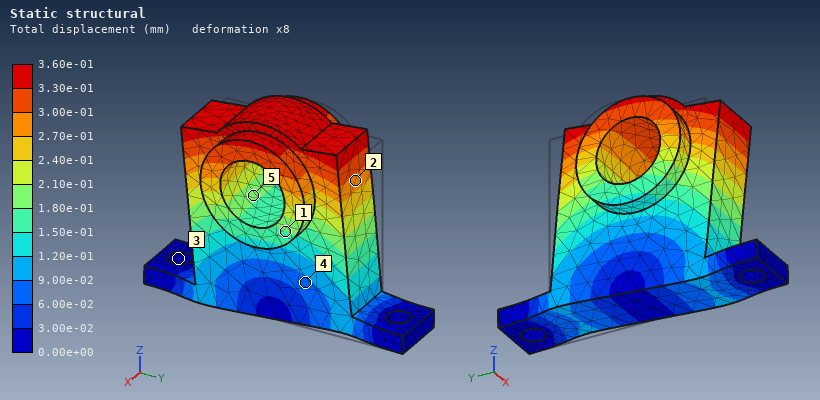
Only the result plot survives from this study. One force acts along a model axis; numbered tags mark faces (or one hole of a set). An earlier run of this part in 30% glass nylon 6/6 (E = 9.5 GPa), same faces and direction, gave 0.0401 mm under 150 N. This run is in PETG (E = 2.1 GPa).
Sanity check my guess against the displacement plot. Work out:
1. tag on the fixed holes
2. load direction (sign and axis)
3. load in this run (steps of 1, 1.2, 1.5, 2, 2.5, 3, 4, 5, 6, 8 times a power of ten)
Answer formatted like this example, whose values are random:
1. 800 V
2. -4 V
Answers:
1. 3
2. -Y
3. 300 N
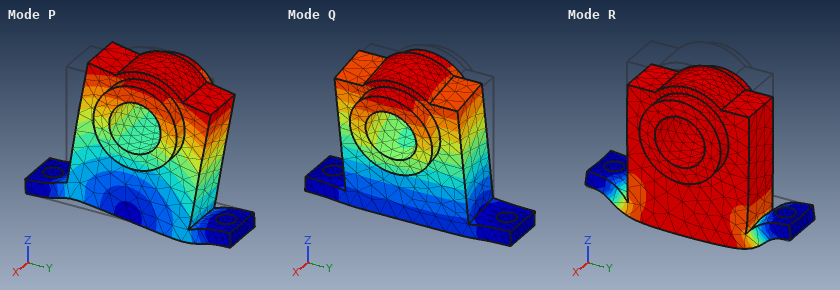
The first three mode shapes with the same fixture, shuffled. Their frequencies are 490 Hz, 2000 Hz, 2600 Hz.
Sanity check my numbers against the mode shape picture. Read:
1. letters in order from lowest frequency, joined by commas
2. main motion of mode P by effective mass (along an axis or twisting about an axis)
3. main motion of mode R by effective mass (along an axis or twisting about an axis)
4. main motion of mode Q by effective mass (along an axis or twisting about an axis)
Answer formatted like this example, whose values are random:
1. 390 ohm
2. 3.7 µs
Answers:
1. Q, P, R
2. along Y
3. along Z
4. along X
